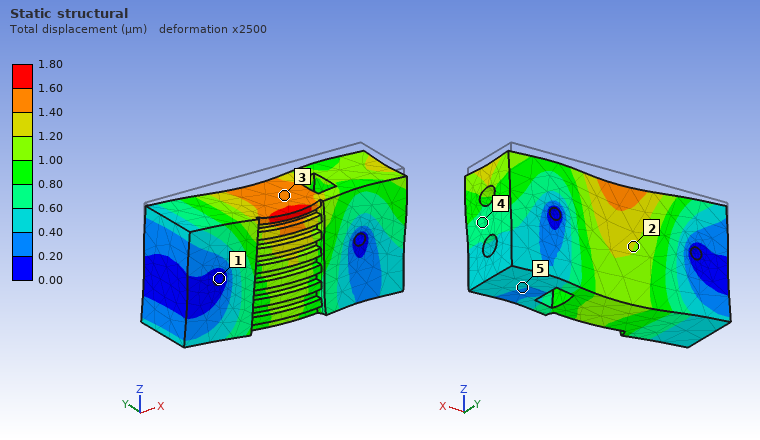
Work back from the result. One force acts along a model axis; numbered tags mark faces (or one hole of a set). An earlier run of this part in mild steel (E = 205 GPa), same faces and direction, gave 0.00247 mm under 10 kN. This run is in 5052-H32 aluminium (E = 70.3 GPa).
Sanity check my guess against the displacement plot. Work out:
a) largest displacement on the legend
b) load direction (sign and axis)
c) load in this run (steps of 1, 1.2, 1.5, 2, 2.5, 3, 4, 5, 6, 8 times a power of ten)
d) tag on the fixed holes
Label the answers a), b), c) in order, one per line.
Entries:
a) 1.80 µm
b) -Z
c) 2.5 kN
d) 1
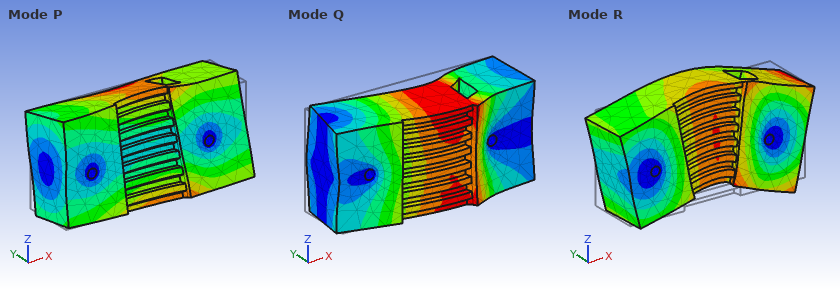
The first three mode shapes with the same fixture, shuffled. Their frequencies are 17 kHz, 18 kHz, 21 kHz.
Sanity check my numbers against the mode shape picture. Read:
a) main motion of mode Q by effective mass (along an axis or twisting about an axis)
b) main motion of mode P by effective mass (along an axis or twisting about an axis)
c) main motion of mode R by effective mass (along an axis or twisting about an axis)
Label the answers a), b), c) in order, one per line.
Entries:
a) along Y
b) twisting about X
c) along Z
